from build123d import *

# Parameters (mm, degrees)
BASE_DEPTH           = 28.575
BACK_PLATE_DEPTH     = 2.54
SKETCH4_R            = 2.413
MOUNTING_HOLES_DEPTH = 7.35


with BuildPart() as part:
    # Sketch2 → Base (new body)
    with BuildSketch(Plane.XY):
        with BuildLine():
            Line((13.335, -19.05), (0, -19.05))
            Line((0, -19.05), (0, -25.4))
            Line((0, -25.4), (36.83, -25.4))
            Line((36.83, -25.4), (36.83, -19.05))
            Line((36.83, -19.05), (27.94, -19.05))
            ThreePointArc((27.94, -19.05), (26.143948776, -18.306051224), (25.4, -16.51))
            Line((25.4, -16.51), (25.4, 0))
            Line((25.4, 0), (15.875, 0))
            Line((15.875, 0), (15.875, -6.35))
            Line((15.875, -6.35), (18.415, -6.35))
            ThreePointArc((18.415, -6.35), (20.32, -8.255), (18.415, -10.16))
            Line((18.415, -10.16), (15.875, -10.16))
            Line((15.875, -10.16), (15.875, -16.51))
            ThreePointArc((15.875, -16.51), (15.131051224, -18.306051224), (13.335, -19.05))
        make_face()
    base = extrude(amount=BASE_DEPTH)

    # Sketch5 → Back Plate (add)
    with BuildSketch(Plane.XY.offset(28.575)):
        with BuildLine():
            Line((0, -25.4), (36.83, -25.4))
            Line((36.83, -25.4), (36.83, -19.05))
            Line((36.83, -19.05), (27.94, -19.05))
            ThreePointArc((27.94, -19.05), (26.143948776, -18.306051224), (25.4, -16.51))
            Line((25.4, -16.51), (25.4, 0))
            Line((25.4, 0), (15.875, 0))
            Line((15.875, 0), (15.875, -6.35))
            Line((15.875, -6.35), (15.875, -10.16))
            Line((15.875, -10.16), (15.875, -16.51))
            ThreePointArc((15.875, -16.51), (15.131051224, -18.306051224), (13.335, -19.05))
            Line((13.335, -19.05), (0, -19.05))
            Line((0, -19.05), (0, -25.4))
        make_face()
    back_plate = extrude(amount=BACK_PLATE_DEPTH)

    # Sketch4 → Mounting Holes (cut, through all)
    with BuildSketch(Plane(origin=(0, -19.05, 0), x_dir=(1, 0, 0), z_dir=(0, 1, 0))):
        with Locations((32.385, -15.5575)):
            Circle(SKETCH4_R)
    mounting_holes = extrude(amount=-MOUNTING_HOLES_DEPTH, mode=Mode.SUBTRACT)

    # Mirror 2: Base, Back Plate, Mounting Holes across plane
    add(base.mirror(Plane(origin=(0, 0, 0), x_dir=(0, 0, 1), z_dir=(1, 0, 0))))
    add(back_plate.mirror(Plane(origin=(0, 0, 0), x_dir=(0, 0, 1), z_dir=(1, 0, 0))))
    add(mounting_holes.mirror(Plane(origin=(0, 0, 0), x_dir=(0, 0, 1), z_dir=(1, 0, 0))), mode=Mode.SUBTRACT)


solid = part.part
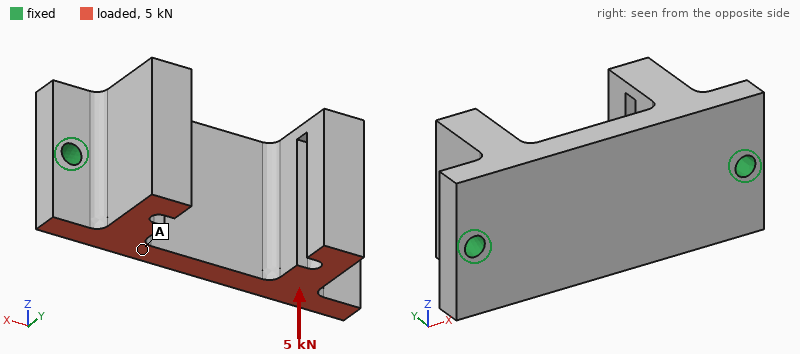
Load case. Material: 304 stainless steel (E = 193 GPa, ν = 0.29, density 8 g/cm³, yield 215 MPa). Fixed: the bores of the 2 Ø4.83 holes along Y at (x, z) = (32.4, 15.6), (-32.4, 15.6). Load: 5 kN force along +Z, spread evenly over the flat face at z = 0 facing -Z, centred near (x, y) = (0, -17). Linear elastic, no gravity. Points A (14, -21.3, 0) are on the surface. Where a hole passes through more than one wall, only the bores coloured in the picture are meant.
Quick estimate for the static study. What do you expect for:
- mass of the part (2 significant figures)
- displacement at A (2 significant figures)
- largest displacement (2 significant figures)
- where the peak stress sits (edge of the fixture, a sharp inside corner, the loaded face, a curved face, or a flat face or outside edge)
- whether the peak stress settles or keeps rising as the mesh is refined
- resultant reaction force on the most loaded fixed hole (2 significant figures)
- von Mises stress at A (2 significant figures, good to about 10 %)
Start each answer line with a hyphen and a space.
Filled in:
- 200 g
- 12 µm
- 24 µm
- edge of the fixture
- keeps rising
- 2.5 kN
- 17 MPa
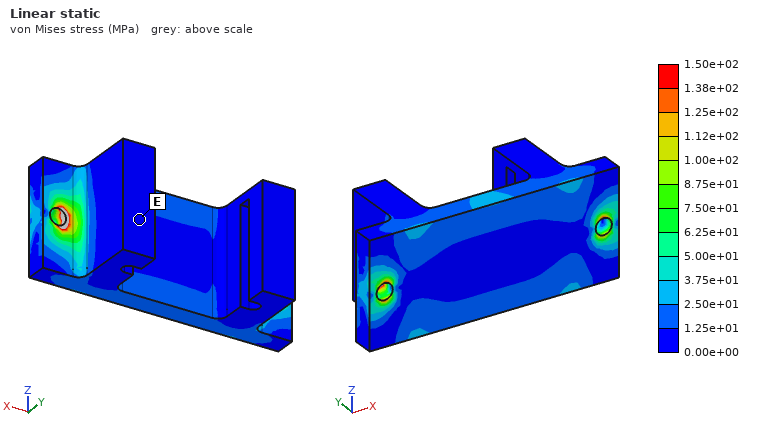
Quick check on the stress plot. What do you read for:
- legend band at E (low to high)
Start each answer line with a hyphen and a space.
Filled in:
- 0.00e+00 to 1.25e+01 MPa
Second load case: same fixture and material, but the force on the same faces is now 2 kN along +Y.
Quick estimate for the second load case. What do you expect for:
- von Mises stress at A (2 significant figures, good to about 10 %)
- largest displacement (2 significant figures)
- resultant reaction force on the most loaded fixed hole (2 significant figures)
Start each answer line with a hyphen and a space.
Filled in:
- 27 MPa
- 32 µm
- 1.0 kN
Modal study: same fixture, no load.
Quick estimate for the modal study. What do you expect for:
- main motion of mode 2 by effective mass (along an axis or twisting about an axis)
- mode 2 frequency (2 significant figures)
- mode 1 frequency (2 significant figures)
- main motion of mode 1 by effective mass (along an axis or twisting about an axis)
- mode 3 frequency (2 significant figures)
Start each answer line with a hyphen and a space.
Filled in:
- along Z
- 5200 Hz
- 4600 Hz
- along Y
- 7600 Hz
